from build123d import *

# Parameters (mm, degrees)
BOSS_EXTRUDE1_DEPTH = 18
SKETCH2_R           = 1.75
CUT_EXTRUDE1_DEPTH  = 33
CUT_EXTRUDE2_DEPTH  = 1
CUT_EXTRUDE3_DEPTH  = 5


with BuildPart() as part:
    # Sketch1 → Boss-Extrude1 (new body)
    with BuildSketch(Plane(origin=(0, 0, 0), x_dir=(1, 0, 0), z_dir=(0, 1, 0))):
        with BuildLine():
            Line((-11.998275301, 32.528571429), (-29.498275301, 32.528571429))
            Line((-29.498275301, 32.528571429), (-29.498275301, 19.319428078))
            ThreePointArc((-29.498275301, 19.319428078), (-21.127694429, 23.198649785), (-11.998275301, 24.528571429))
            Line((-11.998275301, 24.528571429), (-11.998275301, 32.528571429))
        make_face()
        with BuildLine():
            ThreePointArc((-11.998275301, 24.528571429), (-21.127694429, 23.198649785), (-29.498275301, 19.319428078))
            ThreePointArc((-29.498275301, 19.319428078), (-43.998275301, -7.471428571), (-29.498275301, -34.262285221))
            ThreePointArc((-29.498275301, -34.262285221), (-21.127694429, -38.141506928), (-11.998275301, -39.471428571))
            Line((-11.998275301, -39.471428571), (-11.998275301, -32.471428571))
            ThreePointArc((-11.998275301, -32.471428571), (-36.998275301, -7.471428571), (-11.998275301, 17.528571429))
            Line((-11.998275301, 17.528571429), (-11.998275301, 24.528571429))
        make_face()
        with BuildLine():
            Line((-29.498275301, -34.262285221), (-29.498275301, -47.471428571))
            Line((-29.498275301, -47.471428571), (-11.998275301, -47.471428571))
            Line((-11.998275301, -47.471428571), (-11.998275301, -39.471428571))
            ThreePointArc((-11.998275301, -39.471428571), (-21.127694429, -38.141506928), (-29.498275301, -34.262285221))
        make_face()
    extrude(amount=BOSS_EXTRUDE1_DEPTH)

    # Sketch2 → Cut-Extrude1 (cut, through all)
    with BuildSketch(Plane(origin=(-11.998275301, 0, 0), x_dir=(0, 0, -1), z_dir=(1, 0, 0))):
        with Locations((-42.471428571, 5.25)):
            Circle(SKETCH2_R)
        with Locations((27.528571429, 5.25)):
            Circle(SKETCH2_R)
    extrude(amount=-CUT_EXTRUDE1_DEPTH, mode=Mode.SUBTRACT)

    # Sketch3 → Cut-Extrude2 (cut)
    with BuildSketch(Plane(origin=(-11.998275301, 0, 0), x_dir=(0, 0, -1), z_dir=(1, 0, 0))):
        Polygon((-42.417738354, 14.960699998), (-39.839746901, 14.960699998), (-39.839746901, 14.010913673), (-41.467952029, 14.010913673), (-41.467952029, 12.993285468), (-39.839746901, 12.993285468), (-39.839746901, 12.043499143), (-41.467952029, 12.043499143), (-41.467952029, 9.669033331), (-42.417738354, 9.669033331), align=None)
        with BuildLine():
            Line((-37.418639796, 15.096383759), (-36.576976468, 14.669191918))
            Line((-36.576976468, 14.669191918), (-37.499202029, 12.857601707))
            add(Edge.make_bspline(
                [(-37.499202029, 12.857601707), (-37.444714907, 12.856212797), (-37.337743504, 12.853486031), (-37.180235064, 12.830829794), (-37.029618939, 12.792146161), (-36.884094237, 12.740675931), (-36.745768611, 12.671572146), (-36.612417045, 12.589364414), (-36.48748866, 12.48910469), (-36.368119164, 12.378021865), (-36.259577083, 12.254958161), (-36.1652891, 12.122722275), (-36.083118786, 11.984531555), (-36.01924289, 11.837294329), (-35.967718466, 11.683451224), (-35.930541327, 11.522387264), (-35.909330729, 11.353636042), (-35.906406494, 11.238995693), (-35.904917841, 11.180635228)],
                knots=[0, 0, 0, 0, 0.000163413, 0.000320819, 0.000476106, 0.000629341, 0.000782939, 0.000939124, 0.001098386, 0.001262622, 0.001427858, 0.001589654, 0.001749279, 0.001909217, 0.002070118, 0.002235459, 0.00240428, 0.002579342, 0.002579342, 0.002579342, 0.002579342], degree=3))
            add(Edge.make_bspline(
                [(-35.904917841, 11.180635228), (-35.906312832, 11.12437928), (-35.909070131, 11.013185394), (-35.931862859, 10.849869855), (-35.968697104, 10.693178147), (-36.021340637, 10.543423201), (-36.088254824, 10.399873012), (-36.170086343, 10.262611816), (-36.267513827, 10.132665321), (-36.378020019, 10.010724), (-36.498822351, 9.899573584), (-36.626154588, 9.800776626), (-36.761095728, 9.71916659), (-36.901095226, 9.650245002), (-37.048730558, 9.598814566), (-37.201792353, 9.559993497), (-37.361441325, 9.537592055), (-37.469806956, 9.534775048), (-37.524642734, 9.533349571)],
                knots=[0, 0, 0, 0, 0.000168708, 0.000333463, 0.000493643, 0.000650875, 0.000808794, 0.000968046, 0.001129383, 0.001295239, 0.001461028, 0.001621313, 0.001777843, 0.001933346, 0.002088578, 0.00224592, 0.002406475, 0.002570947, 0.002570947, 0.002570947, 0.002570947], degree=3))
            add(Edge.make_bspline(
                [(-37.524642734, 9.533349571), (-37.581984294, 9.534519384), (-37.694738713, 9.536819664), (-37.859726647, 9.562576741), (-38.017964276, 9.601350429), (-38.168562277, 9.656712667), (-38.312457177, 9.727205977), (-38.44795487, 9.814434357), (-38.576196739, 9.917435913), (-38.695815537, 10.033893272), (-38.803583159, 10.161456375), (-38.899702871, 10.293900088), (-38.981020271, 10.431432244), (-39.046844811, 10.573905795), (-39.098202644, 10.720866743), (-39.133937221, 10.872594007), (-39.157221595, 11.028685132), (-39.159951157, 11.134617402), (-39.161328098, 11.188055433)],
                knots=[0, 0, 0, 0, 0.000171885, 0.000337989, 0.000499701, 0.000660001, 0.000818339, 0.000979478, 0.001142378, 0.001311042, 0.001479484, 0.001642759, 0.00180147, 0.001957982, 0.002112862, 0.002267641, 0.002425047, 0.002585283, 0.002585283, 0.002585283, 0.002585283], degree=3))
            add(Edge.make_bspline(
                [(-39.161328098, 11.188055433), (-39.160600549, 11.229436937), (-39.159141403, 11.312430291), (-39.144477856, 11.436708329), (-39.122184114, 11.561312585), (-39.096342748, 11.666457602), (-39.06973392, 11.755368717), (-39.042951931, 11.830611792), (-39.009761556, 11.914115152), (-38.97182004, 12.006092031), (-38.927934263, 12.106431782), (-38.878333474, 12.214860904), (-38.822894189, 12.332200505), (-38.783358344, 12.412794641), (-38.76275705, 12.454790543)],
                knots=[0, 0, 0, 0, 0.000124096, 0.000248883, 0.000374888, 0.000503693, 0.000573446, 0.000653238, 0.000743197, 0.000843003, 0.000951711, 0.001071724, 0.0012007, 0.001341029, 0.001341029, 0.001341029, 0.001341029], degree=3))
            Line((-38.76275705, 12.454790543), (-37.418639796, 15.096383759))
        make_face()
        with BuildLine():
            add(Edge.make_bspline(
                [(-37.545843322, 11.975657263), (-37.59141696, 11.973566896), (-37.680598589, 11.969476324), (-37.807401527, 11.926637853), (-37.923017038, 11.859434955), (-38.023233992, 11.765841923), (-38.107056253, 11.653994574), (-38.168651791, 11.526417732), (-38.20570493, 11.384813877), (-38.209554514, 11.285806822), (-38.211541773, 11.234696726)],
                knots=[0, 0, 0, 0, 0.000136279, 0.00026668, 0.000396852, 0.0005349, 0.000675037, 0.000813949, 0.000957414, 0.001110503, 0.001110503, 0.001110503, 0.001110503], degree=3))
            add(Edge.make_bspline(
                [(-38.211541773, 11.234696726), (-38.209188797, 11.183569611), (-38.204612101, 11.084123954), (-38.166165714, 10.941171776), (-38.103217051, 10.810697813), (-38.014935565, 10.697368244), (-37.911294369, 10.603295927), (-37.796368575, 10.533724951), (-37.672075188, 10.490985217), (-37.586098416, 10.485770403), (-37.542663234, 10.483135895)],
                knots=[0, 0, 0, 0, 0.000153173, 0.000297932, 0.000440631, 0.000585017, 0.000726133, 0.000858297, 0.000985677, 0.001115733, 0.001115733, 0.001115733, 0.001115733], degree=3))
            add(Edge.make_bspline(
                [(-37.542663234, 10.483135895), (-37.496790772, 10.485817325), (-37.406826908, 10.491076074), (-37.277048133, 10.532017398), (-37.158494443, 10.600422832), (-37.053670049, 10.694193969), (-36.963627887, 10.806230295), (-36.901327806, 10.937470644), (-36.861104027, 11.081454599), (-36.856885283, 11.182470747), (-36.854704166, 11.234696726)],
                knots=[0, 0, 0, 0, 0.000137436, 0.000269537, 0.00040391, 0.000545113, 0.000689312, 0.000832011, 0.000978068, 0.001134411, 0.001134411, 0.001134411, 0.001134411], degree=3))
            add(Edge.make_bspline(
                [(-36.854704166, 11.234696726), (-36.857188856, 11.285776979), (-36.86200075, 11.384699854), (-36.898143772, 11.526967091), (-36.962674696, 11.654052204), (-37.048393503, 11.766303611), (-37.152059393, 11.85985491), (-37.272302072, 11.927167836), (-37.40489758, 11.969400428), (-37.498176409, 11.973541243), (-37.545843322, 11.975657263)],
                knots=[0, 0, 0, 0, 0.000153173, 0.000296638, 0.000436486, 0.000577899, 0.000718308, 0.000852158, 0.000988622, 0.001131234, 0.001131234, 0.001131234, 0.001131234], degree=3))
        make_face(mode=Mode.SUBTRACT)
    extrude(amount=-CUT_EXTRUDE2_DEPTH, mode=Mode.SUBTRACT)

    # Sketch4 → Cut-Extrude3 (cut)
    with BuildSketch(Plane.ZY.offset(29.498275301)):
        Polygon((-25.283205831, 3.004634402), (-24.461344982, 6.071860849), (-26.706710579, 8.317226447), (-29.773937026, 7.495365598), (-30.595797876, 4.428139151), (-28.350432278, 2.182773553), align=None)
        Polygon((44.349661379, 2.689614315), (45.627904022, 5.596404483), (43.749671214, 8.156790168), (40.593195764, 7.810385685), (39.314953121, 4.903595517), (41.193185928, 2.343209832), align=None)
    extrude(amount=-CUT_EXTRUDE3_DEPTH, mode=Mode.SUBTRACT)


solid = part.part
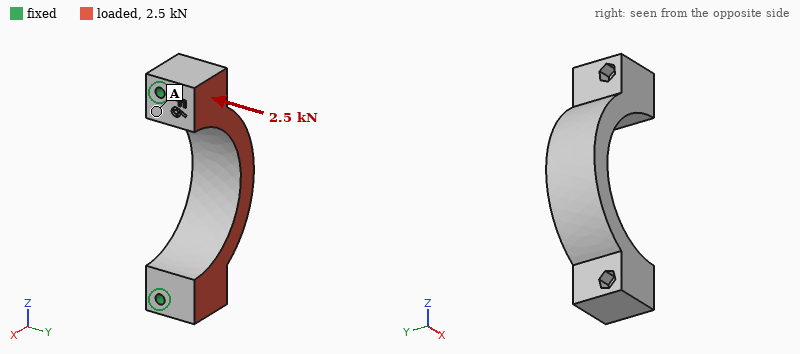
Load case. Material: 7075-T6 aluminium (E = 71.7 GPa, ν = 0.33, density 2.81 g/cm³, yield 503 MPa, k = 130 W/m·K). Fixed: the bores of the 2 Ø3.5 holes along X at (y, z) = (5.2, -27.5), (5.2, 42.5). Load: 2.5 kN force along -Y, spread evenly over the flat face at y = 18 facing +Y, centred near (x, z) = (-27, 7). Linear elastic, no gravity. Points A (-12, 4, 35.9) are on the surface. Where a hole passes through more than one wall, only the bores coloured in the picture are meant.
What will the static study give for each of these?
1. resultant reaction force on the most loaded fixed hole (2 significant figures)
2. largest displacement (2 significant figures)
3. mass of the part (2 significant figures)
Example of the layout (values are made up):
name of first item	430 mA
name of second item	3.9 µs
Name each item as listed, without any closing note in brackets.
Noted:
resultant reaction force on the most loaded fixed hole	1.3 kN
largest displacement	45 µm
mass of the part	47 g
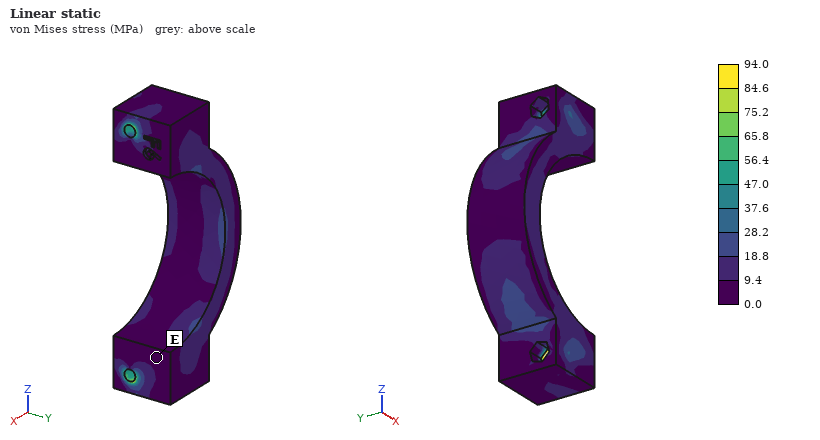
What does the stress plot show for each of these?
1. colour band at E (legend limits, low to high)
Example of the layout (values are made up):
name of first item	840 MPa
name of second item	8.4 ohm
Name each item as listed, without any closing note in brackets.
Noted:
colour band at E	0.0 to 9.4 MPa
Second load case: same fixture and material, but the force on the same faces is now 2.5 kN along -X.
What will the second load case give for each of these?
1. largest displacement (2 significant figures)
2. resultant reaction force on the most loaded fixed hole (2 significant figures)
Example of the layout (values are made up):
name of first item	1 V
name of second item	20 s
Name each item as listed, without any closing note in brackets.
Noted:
largest displacement	38 µm
resultant reaction force on the most loaded fixed hole	1.3 kN
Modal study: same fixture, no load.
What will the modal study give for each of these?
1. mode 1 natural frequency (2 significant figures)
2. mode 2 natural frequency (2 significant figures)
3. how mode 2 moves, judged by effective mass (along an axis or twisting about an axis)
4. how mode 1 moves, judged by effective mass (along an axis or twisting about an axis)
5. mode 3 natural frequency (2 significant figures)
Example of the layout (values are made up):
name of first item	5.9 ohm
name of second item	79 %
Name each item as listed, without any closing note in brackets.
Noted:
mode 1 natural frequency	6600 Hz
mode 2 natural frequency	13 kHz
how mode 2 moves, judged by effective mass	along Z
how mode 1 moves, judged by effective mass	along Y
mode 3 natural frequency	17 kHz
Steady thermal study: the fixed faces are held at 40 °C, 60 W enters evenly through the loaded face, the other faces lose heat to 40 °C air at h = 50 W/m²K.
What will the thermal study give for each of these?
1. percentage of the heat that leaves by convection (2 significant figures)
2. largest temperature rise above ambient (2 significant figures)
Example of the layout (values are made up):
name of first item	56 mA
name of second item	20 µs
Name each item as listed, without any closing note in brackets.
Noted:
percentage of the heat that leaves by convection	4.9 %
largest temperature rise above ambient	24 K
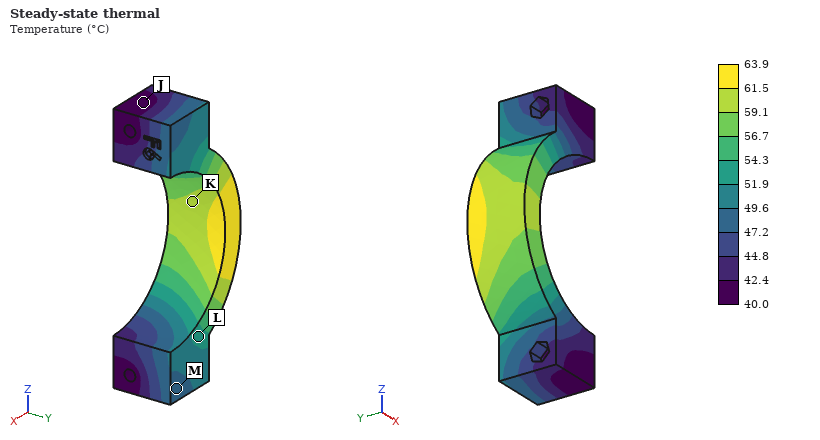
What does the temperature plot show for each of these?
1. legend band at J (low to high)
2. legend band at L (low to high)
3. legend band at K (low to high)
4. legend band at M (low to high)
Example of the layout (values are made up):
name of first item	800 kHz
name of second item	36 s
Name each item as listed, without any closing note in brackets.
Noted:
legend band at J	40.0 to 42.4 °C
legend band at L	51.9 to 54.3 °C
legend band at K	59.1 to 61.5 °C
legend band at M	47.2 to 49.6 °C
